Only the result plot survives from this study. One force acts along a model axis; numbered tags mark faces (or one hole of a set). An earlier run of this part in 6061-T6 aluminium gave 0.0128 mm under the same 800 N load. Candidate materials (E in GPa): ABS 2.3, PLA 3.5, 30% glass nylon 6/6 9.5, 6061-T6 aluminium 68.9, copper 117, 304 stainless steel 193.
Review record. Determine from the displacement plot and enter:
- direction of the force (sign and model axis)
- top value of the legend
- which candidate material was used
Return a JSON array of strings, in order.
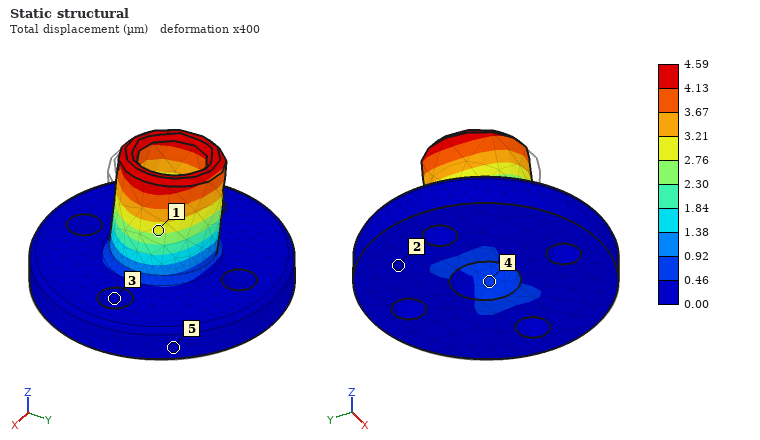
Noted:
["-X", "4.59 µm", "304 stainless steel"]
